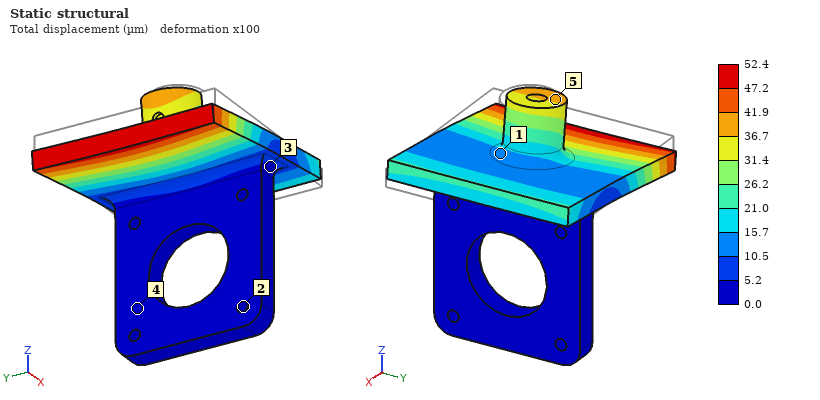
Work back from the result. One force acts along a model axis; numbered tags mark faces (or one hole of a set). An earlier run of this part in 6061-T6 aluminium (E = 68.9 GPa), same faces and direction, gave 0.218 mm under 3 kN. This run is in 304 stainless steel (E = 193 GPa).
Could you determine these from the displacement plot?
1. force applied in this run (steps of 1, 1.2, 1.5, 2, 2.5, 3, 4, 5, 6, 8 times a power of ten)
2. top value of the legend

2 kN
52.4 µm
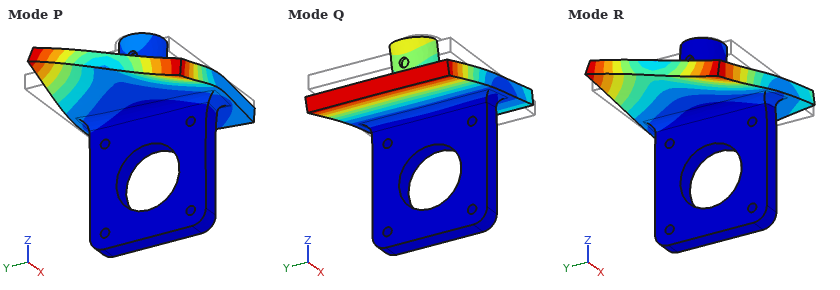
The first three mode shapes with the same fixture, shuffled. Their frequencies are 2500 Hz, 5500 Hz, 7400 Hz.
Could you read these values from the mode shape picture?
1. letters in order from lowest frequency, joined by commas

Q, R, P
